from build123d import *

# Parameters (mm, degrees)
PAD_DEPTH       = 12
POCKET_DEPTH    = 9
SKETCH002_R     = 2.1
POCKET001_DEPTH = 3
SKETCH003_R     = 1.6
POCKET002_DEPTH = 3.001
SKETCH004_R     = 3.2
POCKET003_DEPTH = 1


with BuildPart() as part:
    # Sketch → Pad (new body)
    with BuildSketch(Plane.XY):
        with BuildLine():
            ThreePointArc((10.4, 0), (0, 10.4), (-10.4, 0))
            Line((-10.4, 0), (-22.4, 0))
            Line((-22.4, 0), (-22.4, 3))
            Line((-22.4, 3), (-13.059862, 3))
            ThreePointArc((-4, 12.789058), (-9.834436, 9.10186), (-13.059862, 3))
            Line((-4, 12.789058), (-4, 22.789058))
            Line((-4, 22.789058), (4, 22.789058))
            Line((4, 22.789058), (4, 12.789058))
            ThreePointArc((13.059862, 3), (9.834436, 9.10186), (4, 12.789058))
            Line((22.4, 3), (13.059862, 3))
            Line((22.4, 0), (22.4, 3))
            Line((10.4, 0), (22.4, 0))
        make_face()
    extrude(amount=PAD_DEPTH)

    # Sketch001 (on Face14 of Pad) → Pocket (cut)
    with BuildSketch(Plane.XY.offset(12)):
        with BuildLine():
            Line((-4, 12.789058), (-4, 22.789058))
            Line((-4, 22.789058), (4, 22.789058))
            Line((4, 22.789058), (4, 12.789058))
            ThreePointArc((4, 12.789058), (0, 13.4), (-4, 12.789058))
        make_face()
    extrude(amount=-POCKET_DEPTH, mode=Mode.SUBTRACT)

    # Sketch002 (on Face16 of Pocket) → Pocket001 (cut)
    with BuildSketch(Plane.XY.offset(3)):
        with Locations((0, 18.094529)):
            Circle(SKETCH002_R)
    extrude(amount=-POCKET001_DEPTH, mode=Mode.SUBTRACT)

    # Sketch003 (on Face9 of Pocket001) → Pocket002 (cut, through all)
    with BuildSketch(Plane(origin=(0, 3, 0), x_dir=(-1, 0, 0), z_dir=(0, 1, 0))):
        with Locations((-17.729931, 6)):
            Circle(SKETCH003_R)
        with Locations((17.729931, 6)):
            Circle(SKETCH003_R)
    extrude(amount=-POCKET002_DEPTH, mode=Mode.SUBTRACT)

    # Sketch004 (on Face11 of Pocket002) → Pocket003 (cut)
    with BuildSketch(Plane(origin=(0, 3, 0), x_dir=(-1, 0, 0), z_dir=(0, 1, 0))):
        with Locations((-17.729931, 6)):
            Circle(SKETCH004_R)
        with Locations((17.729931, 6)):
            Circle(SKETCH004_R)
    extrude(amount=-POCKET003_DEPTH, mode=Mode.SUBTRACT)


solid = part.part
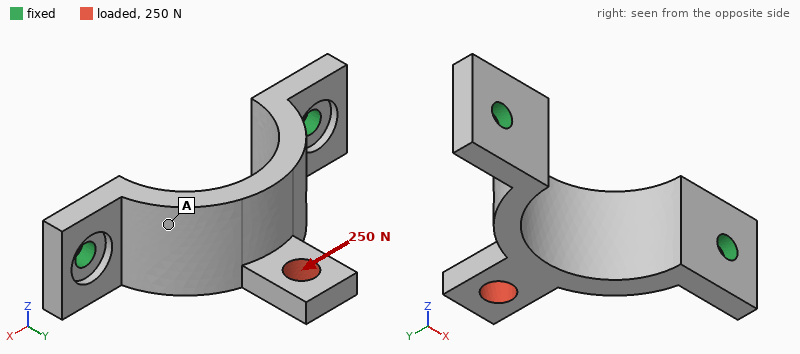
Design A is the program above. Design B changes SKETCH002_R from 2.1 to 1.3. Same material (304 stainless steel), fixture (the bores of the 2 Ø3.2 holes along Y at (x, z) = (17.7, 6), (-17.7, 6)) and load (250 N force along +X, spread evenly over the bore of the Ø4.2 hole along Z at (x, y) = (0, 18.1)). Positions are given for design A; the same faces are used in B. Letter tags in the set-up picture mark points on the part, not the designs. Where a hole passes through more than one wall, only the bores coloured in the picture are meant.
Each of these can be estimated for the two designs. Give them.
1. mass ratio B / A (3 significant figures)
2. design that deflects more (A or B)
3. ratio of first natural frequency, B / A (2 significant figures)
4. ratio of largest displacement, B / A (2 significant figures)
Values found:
1.01
A
0.97
0.87
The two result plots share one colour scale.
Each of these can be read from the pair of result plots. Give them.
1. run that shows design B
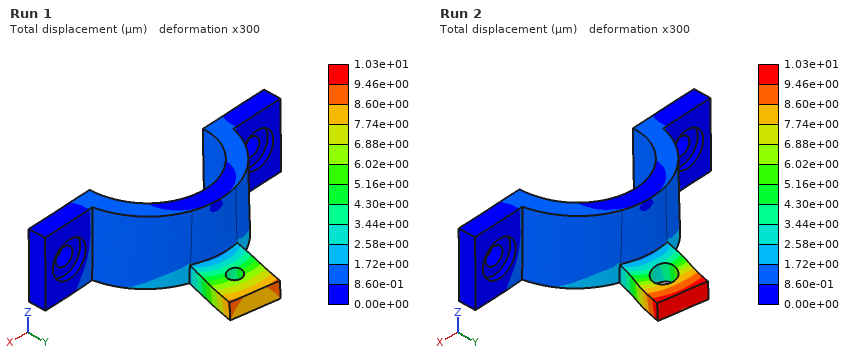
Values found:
Run 1
